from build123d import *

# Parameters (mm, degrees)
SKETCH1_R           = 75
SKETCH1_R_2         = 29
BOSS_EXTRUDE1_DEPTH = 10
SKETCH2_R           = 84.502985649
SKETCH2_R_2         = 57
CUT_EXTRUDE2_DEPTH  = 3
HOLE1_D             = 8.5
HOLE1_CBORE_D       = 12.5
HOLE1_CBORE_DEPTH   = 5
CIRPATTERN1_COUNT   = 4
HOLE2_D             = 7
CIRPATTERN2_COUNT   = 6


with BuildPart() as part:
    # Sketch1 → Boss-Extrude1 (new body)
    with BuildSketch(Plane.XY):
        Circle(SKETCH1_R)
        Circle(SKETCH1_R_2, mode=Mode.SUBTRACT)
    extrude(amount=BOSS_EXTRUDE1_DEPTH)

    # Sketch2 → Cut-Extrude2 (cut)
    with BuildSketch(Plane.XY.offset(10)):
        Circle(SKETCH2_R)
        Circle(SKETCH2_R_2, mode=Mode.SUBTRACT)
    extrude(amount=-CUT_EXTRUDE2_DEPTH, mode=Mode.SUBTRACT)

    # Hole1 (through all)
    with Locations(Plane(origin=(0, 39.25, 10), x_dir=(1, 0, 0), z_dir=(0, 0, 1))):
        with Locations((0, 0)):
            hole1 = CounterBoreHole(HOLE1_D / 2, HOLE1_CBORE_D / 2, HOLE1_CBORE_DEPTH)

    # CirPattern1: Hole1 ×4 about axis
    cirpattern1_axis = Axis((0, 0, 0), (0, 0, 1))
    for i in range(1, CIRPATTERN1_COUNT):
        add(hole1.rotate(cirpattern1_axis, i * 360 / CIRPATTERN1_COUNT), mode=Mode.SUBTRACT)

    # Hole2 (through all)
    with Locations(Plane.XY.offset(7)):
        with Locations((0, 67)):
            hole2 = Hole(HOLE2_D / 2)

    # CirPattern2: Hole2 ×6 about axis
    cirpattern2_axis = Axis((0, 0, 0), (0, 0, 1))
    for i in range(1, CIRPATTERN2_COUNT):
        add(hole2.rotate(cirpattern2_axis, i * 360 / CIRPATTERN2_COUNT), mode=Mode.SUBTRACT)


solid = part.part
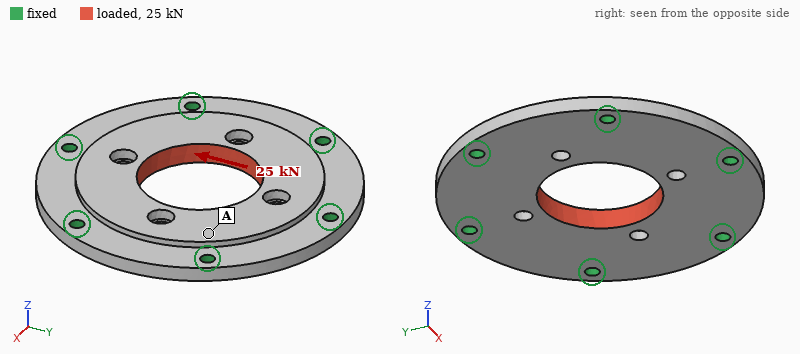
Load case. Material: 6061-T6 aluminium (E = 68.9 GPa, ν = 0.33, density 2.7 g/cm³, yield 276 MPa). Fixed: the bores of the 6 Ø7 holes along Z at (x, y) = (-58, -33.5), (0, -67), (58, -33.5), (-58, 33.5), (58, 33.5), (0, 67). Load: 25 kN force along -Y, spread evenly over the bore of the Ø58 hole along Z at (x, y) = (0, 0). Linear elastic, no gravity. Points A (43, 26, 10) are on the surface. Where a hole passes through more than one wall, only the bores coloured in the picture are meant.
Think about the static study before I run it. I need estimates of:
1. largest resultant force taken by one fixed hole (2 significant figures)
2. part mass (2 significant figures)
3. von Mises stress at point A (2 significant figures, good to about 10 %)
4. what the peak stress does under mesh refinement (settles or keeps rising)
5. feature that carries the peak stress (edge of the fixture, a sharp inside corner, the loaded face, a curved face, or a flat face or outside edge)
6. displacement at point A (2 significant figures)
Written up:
5.8 kN
330 g
10 MPa
keeps rising
edge of the fixture
8.1 µm
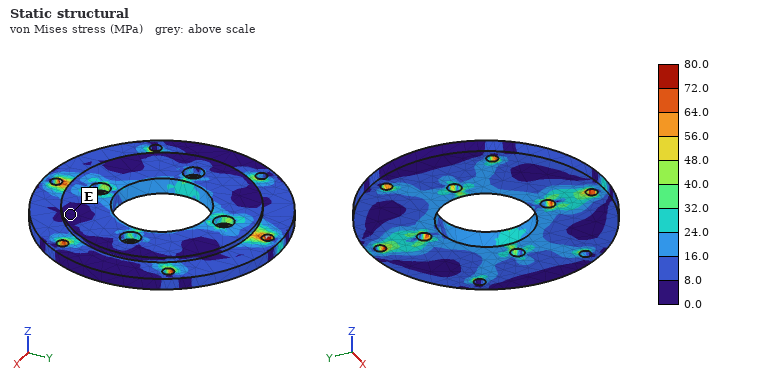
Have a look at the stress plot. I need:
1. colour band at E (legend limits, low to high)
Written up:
0.0 to 8.0 MPa
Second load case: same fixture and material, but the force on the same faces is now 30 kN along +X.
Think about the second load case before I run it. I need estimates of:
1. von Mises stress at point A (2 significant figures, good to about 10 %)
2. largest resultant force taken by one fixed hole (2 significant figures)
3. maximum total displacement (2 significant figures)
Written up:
20 MPa
6.2 kN
28 µm
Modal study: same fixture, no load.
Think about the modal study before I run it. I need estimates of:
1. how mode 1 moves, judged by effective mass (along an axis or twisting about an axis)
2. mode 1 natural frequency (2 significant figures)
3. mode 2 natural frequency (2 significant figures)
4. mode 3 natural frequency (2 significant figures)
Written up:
along Z
4300 Hz
6400 Hz
6500 Hz
